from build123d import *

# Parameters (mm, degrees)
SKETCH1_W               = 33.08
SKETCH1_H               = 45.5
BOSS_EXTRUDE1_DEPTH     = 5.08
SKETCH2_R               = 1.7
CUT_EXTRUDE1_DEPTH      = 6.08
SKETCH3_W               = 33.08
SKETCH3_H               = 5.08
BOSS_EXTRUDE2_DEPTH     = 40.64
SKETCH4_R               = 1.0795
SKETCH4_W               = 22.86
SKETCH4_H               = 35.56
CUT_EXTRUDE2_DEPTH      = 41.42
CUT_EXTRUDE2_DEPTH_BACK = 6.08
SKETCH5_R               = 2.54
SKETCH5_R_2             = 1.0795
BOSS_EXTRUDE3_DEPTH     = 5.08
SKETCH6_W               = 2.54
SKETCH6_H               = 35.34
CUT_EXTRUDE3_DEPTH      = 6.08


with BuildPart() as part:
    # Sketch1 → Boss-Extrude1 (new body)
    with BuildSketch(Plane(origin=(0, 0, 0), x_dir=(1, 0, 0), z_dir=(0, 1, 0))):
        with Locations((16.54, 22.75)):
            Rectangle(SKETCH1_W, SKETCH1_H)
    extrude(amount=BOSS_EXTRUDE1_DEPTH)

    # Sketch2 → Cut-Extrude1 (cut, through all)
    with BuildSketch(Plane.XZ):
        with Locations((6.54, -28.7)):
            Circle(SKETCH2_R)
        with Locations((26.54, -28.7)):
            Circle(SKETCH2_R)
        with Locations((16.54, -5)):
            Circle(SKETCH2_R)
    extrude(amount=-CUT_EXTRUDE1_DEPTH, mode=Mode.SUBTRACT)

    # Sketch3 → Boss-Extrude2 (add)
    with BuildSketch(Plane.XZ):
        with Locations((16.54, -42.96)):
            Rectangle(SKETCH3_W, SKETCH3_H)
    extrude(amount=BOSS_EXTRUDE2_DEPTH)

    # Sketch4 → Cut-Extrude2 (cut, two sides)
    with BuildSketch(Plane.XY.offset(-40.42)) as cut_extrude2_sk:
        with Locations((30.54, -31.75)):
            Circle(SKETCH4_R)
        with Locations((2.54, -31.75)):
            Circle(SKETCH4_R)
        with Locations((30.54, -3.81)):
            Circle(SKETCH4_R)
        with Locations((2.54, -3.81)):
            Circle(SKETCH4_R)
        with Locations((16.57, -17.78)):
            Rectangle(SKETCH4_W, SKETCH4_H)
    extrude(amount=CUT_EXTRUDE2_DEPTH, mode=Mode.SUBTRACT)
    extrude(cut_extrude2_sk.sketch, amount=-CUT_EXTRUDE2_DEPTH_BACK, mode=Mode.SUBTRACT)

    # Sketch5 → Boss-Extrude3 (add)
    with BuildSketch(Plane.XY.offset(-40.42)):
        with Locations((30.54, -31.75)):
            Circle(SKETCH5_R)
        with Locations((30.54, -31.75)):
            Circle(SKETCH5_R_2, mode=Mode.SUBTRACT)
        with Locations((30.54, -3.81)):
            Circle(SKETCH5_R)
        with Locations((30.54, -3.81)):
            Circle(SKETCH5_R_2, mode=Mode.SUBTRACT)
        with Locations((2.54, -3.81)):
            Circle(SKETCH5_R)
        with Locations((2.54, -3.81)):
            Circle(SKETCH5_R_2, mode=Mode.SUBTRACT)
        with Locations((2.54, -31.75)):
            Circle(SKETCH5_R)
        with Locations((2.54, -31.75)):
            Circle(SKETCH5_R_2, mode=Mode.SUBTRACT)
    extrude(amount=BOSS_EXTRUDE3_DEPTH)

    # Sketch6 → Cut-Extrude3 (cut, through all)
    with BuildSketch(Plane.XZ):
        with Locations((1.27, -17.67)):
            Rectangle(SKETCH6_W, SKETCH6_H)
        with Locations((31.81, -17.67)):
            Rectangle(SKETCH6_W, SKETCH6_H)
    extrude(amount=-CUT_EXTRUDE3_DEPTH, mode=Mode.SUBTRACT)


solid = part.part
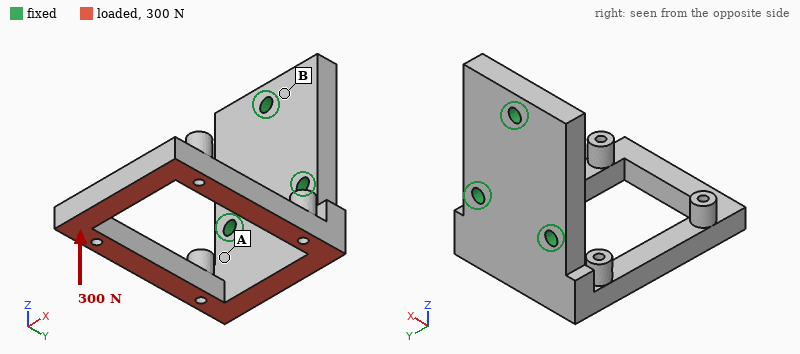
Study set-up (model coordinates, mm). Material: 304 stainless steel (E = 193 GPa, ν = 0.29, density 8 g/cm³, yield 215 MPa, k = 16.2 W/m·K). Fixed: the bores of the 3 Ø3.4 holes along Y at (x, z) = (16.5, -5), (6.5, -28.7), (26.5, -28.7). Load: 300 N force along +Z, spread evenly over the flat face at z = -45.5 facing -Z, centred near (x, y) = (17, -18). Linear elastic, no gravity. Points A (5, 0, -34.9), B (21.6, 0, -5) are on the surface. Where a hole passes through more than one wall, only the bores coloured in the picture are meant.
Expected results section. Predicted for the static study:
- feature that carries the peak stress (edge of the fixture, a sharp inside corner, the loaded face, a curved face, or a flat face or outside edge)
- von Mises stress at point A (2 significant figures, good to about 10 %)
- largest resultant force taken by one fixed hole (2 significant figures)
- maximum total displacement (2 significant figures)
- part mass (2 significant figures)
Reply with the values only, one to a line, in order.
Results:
the loaded face
64 MPa
150 N
0.22 mm
76 g
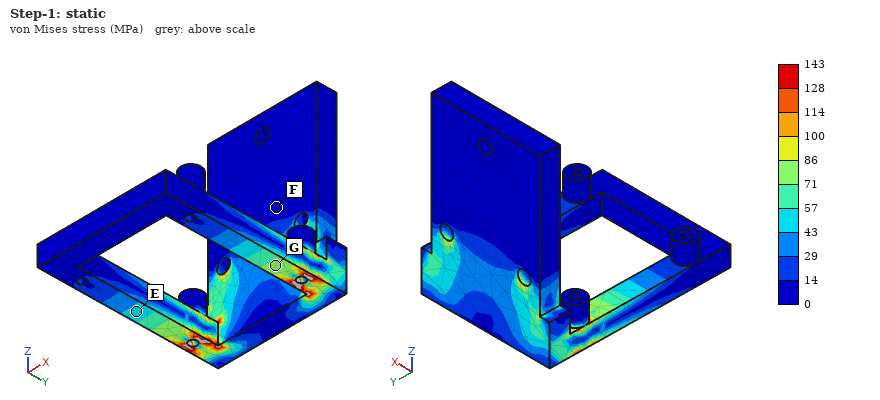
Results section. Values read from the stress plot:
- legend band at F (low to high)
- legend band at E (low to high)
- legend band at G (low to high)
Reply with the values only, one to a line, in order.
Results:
0 to 14 MPa
43 to 57 MPa
71 to 86 MPa
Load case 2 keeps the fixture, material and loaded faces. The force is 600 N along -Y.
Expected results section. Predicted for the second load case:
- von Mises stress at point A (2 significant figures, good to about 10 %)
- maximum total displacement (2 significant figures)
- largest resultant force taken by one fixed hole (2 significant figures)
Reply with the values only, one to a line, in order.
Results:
59 MPa
0.11 mm
340 N
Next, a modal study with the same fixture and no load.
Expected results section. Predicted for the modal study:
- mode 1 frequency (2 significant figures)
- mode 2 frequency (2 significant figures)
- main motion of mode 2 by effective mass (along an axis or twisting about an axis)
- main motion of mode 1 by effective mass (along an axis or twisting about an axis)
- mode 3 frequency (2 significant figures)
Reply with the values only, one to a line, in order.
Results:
1200 Hz
2000 Hz
along X
along Z
3200 Hz
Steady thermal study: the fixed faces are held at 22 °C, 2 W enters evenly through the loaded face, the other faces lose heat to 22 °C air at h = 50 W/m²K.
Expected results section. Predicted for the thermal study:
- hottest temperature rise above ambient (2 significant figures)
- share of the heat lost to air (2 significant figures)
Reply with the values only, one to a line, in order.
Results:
15 K
67 %
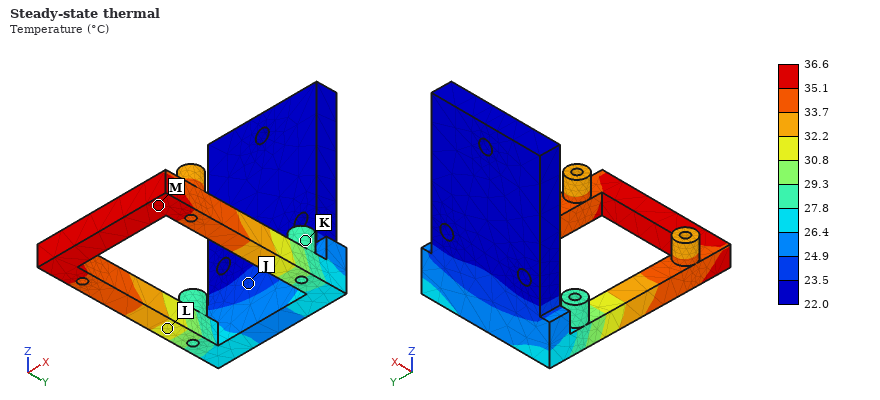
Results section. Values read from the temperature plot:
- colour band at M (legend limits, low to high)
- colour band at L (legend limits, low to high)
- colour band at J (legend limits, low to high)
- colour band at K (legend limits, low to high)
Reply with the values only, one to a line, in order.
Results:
35.1 to 36.6 °C
30.8 to 32.2 °C
23.5 to 24.9 °C
27.8 to 29.3 °C
